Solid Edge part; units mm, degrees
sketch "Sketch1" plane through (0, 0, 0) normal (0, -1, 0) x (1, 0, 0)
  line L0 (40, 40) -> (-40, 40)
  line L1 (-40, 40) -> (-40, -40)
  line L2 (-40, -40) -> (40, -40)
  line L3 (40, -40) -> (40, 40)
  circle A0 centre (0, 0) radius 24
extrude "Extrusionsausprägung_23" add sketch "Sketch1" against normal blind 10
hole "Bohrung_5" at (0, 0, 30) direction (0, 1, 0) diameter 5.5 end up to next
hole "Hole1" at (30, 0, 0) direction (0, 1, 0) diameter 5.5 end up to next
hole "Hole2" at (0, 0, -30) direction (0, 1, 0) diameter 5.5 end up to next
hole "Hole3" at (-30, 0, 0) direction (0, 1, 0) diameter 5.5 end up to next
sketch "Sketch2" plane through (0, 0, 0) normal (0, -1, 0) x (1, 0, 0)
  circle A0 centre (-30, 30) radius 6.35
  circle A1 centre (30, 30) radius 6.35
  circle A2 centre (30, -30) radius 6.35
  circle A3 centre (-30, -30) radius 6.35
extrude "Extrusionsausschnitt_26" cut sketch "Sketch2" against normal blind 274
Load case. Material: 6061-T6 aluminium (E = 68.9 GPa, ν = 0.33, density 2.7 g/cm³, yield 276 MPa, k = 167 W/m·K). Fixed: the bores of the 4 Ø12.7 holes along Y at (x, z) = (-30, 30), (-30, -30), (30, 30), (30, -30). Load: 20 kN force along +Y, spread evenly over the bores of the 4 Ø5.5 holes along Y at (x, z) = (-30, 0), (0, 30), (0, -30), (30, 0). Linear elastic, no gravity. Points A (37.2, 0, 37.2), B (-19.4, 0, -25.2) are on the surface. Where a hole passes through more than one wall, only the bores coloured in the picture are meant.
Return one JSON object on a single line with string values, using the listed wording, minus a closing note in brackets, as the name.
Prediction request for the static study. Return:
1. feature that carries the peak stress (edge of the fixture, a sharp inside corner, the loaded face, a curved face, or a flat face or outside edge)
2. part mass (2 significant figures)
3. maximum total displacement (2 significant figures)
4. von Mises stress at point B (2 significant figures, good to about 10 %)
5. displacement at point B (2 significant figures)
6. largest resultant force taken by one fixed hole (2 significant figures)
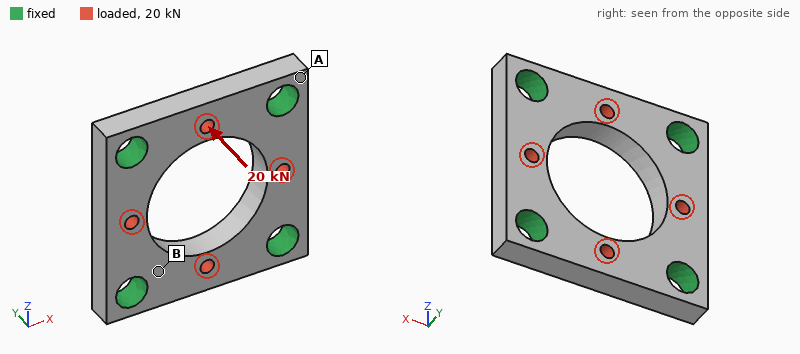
{"feature that carries the peak stress": "the loaded face", "part mass": "110 g", "maximum total displacement": "52 µm", "von Mises stress at point B": "53 MPa", "displacement at point B": "12 µm", "largest resultant force taken by one fixed hole": "5.0 kN"}
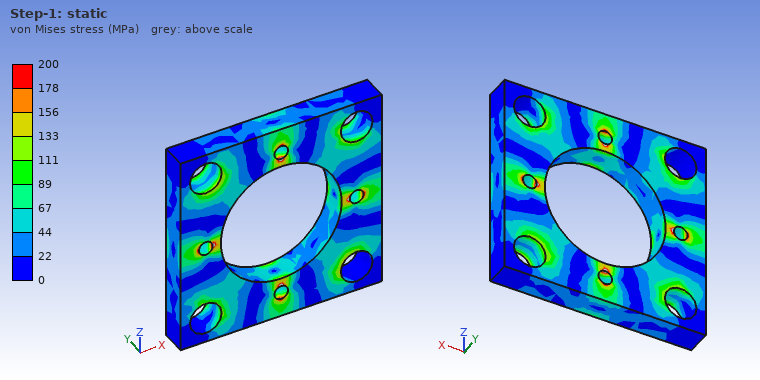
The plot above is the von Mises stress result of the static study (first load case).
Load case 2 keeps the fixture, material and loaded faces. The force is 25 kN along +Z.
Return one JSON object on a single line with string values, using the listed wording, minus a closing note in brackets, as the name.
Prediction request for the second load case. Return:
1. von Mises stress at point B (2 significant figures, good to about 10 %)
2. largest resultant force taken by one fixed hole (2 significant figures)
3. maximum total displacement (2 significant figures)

{"von Mises stress at point B": "23 MPa", "largest resultant force taken by one fixed hole": "6.3 kN", "maximum total displacement": "32 µm"}
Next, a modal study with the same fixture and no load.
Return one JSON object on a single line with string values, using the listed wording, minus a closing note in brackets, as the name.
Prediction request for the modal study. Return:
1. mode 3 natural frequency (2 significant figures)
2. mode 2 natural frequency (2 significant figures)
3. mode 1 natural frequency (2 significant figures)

{"mode 3 natural frequency": "18 kHz", "mode 2 natural frequency": "18 kHz", "mode 1 natural frequency": "17 kHz"}
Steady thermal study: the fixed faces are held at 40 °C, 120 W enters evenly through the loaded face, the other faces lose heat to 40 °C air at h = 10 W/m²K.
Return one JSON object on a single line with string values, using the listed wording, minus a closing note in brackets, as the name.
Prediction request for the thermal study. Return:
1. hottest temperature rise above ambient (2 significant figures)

{"hottest temperature rise above ambient": "13 K"}
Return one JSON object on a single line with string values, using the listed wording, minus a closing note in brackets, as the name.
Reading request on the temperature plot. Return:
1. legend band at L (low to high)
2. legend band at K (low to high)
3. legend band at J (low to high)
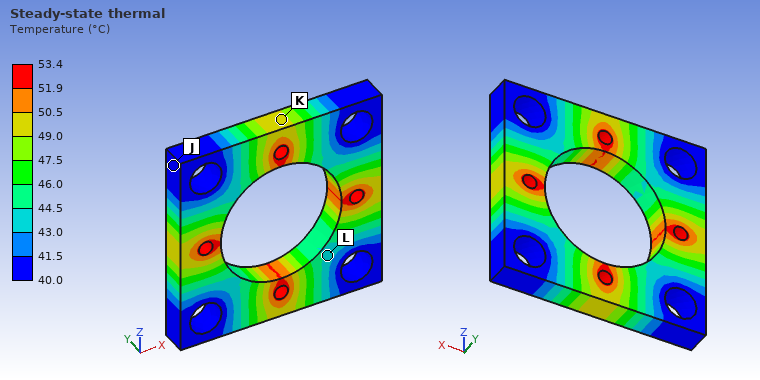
{"legend band at L": "43.0 to 44.5 °C", "legend band at K": "49.0 to 50.5 °C", "legend band at J": "40.0 to 41.5 °C"}
